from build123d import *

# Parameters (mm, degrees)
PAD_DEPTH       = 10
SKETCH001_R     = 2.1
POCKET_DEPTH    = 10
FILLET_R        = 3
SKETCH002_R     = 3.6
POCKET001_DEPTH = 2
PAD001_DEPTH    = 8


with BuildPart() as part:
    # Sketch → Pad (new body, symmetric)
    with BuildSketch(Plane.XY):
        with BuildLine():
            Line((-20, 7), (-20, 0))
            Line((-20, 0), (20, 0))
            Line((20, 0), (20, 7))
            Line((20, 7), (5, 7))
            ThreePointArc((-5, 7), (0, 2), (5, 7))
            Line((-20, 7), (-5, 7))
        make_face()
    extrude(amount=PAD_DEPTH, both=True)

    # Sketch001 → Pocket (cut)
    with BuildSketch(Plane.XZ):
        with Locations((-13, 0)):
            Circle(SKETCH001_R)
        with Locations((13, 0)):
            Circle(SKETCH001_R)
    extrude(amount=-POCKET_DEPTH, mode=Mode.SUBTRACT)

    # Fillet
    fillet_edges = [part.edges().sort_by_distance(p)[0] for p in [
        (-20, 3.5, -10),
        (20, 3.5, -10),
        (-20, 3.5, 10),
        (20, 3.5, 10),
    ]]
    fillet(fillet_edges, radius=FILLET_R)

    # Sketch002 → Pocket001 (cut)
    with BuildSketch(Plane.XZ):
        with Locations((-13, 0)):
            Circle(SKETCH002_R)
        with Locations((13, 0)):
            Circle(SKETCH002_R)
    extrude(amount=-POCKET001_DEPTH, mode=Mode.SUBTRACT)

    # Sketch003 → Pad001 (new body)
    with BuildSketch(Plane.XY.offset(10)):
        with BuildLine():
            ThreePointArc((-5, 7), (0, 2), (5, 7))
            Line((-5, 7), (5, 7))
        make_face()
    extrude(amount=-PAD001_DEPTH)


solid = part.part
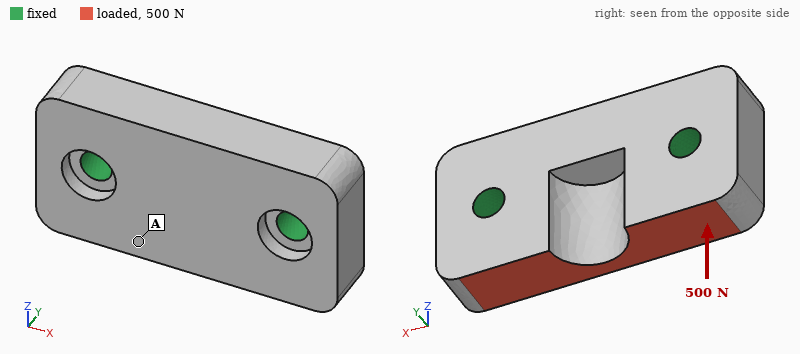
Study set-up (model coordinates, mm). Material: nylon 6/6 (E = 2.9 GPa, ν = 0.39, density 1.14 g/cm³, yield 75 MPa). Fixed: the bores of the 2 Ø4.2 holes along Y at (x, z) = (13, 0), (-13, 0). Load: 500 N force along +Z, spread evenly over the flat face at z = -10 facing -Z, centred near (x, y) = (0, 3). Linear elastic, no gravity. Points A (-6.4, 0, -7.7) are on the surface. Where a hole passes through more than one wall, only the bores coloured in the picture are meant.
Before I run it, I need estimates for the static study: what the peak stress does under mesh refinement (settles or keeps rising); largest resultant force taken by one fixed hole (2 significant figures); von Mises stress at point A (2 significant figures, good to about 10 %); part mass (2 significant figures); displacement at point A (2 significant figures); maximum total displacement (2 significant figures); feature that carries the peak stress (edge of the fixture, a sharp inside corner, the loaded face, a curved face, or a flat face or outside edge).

keeps rising
250 N
2.4 MPa
5.4 g
28 µm
42 µm
edge of the fixture
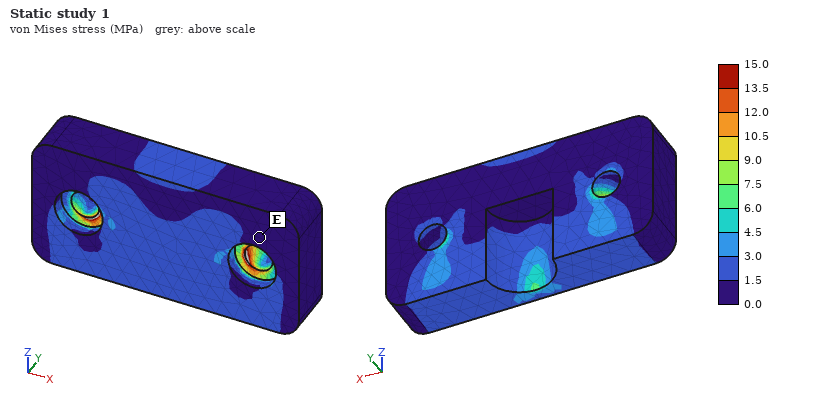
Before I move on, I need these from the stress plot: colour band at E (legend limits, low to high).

0.0 to 1.5 MPa
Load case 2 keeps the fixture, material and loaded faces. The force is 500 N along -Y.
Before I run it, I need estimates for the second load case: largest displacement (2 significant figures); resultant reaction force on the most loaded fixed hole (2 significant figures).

0.22 mm
260 N
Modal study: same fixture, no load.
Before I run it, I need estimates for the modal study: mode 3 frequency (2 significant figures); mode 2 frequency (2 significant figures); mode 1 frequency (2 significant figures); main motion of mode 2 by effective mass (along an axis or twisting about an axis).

11 kHz
9700 Hz
7700 Hz
along Y
